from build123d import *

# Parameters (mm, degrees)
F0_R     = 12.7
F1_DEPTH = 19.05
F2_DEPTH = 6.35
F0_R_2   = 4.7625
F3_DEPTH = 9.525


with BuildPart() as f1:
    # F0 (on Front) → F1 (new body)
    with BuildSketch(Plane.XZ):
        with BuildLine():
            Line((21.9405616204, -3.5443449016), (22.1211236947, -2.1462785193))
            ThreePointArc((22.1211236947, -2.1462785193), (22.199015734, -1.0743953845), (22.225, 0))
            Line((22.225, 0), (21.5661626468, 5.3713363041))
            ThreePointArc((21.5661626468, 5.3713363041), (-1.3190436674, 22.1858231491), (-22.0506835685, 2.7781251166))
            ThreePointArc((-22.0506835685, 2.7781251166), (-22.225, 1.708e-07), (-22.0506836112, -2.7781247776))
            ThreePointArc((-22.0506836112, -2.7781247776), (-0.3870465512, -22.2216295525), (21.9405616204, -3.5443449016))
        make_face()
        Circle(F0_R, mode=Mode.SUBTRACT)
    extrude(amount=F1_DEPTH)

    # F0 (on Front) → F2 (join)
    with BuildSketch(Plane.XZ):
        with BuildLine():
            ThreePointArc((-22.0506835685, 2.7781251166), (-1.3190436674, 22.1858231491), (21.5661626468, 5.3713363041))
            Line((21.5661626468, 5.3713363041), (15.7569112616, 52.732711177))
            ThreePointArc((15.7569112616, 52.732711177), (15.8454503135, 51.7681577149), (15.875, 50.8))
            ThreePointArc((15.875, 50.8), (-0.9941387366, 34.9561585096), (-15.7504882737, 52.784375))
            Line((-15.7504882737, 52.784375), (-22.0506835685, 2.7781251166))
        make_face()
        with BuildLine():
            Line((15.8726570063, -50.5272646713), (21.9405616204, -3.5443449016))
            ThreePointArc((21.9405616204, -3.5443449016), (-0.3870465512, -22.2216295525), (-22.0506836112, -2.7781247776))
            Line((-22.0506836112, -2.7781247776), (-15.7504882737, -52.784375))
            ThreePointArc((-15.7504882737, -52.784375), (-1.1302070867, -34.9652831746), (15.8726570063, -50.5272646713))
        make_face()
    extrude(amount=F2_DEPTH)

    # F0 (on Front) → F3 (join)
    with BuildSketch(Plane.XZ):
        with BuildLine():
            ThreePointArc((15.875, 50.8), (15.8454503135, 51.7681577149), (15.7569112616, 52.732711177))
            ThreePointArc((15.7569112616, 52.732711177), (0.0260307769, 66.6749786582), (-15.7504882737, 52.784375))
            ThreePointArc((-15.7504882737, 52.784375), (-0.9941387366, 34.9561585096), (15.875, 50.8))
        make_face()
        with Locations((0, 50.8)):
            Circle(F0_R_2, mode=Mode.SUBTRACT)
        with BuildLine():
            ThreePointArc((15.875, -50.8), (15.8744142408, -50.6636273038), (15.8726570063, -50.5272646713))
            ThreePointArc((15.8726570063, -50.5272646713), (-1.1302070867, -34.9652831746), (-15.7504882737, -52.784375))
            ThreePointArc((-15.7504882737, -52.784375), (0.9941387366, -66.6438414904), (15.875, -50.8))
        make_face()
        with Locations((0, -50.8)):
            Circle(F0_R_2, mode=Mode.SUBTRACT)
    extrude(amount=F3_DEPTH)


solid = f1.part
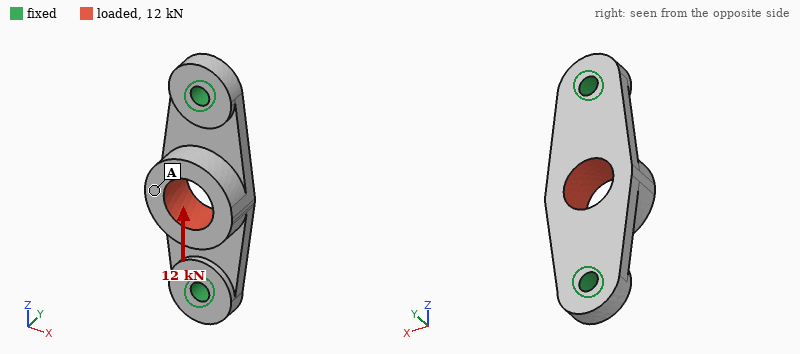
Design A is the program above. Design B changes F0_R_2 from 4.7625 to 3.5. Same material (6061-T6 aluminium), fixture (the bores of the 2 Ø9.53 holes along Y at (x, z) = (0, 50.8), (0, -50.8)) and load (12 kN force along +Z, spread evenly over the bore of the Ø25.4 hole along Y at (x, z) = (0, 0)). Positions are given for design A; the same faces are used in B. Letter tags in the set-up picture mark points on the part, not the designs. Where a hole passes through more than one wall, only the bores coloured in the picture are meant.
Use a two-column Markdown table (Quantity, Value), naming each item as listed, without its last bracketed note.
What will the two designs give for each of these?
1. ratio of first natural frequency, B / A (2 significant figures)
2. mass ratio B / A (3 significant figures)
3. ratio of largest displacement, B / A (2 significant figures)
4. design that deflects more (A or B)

| Quantity | Value |
|---|---|
| ratio of first natural frequency, B / A | 0.97 |
| mass ratio B / A | 1.01 |
| ratio of largest displacement, B / A | 1.1 |
| design that deflects more | B |
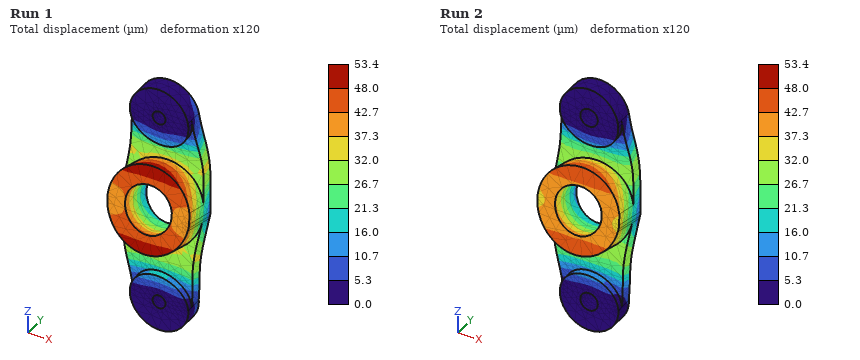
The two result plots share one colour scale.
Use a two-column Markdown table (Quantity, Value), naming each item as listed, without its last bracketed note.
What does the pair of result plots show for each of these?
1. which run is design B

| Quantity | Value |
|---|---|
| which run is design B | Run 1 |
